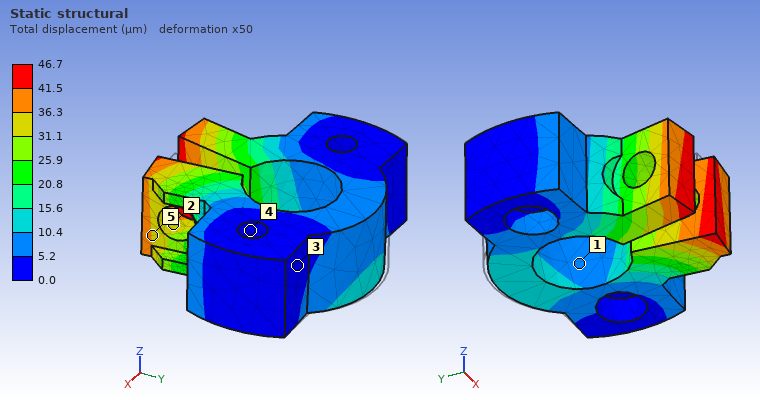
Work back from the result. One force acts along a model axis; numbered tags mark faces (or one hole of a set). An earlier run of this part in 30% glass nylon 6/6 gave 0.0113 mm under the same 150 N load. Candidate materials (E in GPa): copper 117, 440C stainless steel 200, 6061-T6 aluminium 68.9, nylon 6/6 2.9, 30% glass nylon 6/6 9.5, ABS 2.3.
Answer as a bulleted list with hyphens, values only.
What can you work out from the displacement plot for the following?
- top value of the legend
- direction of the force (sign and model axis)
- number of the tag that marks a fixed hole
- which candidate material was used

- 46.7 µm
- -Y
- 4
- ABS
